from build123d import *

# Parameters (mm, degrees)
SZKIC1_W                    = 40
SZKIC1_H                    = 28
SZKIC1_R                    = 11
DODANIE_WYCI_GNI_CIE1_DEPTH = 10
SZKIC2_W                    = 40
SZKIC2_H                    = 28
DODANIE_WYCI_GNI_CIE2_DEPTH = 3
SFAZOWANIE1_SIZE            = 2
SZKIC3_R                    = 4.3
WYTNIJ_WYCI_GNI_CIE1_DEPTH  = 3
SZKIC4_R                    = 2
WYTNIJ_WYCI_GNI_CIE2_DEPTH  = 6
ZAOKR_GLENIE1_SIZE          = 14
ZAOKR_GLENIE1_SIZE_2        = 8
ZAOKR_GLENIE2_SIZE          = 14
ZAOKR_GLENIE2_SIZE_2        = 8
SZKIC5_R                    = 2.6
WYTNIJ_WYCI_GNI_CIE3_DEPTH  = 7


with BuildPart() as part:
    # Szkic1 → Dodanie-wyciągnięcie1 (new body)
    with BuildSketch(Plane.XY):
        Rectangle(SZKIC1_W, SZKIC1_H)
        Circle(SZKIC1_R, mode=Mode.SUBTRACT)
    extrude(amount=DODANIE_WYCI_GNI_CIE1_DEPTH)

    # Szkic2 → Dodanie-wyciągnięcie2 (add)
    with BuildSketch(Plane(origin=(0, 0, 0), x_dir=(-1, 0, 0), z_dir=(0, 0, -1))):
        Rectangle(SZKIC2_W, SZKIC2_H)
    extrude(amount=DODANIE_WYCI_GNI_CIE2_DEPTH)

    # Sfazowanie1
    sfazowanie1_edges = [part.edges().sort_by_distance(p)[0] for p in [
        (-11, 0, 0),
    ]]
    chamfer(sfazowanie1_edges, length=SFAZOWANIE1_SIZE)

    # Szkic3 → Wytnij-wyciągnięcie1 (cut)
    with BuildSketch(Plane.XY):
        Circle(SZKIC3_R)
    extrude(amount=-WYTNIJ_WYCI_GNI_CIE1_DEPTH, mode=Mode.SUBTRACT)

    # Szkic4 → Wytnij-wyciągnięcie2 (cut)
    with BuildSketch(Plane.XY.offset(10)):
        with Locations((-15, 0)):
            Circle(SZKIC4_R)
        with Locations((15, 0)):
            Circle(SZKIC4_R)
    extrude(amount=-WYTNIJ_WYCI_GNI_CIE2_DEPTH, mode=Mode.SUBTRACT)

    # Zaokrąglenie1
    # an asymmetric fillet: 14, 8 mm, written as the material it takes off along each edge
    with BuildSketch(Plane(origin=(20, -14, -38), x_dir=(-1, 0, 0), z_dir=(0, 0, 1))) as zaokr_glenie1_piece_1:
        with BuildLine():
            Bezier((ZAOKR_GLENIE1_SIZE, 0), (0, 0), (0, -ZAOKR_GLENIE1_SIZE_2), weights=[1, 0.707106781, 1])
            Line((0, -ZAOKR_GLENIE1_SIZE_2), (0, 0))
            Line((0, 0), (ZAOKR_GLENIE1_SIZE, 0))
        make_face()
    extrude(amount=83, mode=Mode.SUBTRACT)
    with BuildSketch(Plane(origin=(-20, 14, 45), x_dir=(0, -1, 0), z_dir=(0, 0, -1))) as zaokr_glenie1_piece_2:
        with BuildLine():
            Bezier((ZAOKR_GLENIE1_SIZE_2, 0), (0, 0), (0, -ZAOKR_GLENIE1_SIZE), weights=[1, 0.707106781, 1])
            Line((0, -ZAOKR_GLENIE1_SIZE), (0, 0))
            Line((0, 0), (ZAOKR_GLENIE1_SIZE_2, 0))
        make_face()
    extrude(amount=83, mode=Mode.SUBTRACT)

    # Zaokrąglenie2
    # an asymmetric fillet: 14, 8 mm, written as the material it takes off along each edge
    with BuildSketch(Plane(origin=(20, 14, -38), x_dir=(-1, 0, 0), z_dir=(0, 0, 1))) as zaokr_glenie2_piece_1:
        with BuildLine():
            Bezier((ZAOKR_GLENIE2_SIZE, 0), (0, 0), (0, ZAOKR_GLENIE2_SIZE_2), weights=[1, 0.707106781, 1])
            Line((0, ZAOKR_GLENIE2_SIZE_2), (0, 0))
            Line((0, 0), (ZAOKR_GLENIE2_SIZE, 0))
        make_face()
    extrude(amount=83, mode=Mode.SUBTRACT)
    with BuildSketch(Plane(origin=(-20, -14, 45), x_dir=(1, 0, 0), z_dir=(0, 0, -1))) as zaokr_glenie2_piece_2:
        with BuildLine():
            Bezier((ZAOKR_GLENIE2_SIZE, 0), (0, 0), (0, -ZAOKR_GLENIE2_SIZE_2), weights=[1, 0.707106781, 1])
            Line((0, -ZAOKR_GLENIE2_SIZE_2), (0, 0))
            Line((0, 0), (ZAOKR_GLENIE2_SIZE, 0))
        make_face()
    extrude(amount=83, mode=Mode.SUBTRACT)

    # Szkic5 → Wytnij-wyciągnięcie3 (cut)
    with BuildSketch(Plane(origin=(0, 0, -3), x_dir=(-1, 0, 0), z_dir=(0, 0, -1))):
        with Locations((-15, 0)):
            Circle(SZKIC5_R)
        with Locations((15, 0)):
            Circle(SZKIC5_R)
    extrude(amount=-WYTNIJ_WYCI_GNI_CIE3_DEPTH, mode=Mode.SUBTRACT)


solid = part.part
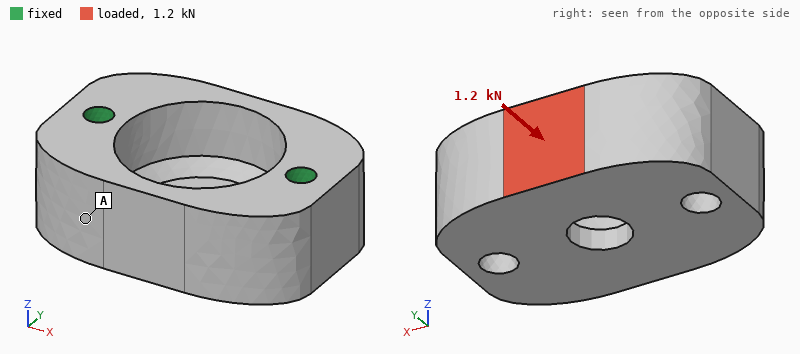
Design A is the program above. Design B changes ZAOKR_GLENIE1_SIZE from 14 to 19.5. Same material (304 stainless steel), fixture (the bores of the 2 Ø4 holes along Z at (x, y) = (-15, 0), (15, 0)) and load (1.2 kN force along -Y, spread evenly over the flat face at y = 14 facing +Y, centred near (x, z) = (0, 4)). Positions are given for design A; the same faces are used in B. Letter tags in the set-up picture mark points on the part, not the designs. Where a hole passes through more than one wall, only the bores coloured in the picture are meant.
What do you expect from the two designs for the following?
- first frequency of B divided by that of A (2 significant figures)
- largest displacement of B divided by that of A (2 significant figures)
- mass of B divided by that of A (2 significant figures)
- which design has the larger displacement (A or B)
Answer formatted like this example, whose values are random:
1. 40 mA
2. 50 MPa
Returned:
1. 1.0
2. 1.1
3. 0.97
4. B
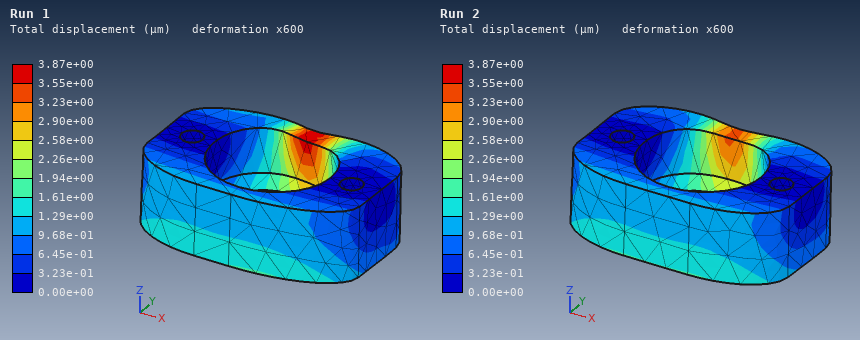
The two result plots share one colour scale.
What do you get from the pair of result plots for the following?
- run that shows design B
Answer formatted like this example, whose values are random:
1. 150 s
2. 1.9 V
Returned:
1. Run 1
